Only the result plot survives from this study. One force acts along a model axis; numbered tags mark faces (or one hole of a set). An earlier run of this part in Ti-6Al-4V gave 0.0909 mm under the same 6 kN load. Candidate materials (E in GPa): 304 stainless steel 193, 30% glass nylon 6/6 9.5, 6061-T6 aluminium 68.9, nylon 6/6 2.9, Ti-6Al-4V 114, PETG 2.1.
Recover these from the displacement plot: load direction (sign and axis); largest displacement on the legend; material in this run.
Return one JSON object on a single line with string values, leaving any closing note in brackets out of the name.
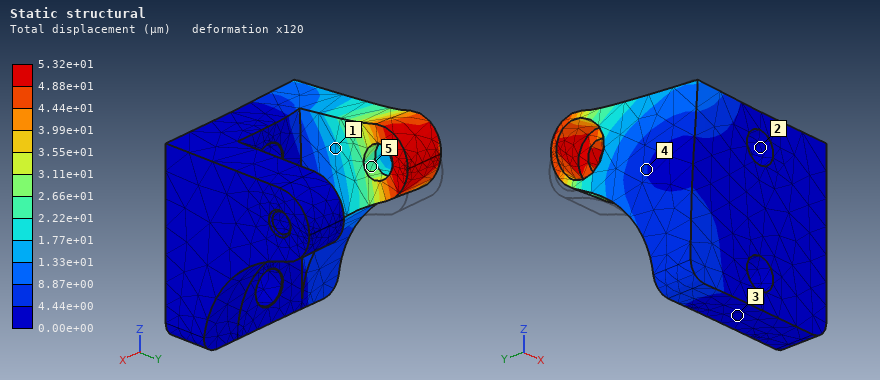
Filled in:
{"load direction": "+Z", "largest displacement on the legend": "5.32e+01 µm", "material in this run": "304 stainless steel"}
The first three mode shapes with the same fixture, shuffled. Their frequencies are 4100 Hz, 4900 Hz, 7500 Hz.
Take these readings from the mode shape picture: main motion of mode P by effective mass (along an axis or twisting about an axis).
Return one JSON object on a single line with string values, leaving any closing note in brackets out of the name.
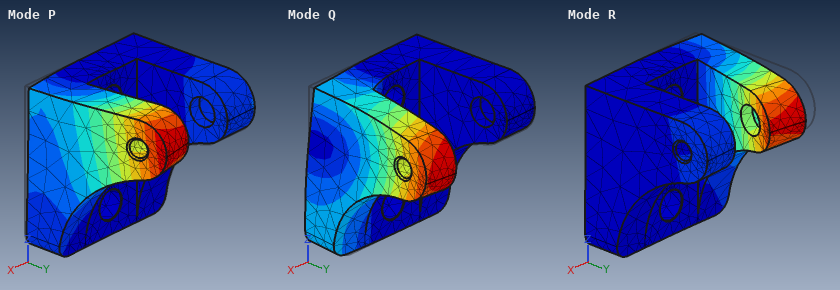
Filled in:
{"main motion of mode P by effective mass": "along X"}
